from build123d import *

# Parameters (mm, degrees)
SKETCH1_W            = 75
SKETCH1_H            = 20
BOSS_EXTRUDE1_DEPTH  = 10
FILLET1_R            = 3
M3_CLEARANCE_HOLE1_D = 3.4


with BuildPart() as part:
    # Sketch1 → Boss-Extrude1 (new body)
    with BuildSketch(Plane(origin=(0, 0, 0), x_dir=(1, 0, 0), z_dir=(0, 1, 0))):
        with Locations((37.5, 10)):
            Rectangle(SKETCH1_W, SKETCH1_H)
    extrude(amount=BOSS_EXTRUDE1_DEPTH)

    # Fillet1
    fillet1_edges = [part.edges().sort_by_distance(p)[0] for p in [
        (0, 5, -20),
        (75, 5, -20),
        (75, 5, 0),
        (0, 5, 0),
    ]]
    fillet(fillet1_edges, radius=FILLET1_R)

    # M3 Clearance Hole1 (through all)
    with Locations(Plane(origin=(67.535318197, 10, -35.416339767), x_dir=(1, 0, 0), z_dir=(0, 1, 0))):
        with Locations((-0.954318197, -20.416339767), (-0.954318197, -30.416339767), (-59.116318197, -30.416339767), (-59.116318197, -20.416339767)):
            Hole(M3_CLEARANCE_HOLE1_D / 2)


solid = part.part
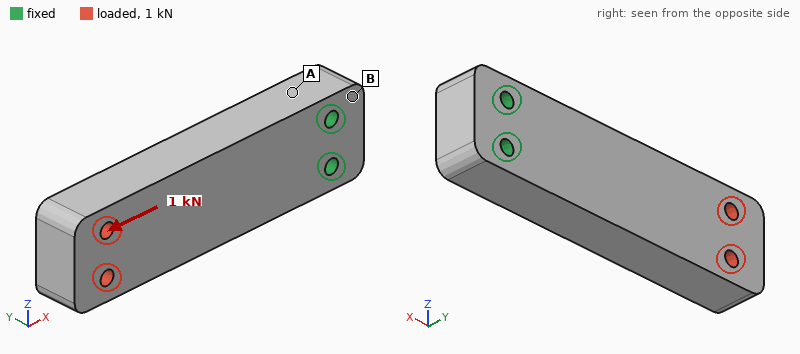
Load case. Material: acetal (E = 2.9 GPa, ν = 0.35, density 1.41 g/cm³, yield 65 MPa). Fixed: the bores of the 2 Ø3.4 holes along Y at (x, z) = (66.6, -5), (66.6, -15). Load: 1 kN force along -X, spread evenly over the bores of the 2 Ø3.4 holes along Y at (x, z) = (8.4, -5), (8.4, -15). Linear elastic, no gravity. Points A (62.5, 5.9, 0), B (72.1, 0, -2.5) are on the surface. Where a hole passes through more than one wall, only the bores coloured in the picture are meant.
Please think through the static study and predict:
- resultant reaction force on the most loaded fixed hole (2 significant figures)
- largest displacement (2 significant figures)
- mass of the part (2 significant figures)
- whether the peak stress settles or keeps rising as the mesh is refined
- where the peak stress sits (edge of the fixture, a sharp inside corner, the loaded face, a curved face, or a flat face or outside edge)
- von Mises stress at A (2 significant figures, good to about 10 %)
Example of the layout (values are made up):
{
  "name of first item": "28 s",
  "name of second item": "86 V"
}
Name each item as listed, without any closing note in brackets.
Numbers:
{
  "resultant reaction force on the most loaded fixed hole": "510 N",
  "largest displacement": "0.11 mm",
  "mass of the part": "21 g",
  "whether the peak stress settles or keeps rising as the mesh is refined": "keeps rising",
  "where the peak stress sits": "edge of the fixture",
  "von Mises stress at A": "3.2 MPa"
}
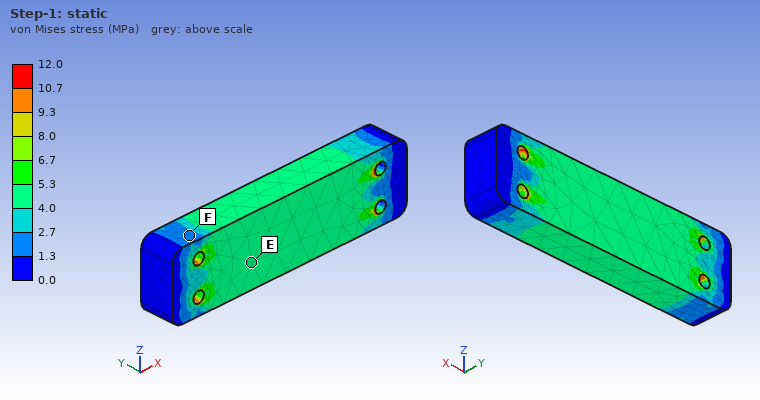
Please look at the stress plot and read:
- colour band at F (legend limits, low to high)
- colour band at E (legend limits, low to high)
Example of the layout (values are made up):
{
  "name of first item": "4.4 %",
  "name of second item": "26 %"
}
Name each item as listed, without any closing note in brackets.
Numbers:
{
  "colour band at F": "1.3 to 2.7 MPa",
  "colour band at E": "4.0 to 5.3 MPa"
}
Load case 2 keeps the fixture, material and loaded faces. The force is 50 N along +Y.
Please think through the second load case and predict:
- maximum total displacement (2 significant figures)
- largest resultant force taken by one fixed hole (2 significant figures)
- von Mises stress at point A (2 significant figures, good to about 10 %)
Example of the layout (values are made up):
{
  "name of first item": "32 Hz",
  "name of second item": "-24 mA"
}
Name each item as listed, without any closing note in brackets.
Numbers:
{
  "maximum total displacement": "0.83 mm",
  "largest resultant force taken by one fixed hole": "25 N",
  "von Mises stress at point A": "1.8 MPa"
}
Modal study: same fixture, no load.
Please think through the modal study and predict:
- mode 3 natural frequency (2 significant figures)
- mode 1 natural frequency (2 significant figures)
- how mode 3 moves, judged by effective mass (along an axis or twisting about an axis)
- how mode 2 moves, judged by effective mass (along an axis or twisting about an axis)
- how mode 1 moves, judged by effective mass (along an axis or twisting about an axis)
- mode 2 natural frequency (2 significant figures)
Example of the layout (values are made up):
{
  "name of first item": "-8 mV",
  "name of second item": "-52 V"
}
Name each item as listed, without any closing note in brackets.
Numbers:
{
  "mode 3 natural frequency": "2600 Hz",
  "mode 1 natural frequency": "530 Hz",
  "how mode 3 moves, judged by effective mass": "twisting about X",
  "how mode 2 moves, judged by effective mass": "along Z",
  "how mode 1 moves, judged by effective mass": "along Y",
  "mode 2 natural frequency": "970 Hz"
}
